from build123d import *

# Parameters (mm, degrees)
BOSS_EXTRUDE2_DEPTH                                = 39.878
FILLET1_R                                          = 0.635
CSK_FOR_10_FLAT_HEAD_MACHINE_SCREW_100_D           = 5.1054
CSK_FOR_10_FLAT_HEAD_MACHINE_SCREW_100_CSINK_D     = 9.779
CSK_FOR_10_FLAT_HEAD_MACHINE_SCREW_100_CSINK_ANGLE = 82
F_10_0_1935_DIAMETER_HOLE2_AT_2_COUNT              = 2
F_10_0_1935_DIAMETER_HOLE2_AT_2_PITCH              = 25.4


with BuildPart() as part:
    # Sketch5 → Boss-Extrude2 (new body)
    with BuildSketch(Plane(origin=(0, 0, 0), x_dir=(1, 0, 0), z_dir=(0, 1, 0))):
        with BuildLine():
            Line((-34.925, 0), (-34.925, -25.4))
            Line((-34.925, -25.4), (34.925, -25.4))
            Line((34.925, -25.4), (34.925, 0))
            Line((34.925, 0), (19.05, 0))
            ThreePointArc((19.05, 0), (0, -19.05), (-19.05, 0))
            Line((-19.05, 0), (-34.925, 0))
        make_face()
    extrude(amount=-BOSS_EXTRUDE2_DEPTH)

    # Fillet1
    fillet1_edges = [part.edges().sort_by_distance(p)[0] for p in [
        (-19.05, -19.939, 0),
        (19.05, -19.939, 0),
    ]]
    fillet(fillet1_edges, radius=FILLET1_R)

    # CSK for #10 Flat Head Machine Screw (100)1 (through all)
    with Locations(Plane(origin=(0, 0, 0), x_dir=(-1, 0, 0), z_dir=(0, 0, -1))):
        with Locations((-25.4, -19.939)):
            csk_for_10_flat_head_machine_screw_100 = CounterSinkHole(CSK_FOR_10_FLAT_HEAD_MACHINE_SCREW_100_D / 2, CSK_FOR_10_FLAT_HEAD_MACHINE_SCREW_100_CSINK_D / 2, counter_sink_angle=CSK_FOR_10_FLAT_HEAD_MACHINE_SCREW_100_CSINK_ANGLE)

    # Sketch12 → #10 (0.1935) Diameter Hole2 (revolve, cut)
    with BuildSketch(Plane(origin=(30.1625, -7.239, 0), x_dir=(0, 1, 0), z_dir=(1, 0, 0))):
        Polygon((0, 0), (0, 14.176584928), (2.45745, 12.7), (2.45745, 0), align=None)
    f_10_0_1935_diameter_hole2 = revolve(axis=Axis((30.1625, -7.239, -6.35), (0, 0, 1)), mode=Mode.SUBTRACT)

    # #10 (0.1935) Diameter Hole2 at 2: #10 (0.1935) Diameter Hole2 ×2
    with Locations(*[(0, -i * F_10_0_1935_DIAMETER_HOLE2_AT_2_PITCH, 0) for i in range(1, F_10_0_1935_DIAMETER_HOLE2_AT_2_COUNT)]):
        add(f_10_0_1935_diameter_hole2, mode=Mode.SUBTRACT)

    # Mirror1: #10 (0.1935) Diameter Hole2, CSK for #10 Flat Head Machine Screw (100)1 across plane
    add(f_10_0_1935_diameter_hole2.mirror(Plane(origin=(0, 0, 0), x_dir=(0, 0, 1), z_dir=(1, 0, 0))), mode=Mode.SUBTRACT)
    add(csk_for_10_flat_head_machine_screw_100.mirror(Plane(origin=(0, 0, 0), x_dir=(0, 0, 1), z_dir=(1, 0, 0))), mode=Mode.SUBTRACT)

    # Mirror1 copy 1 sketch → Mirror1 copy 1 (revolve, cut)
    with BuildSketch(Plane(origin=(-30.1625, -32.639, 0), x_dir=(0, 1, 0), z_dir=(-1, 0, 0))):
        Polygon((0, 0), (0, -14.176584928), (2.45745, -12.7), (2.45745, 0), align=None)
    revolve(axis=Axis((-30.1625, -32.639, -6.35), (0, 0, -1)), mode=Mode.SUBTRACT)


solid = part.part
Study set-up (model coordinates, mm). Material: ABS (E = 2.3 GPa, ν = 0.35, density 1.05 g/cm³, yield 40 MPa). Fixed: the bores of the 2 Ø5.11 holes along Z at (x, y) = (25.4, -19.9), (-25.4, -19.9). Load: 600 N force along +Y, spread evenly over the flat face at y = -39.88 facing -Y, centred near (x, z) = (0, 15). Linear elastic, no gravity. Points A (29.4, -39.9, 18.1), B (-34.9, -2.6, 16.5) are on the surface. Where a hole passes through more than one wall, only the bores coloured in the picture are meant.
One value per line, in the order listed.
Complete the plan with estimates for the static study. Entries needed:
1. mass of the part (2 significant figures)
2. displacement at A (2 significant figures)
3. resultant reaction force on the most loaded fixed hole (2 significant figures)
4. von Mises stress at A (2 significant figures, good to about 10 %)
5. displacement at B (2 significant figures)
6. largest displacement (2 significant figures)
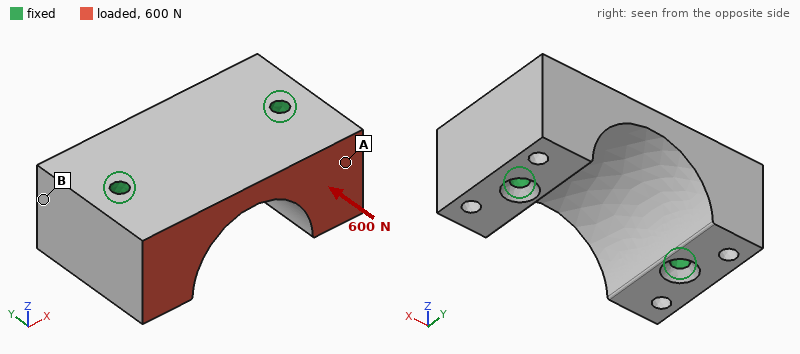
48 g
5.1 µm
300 N
0.56 MPa
2.1 µm
12 µm
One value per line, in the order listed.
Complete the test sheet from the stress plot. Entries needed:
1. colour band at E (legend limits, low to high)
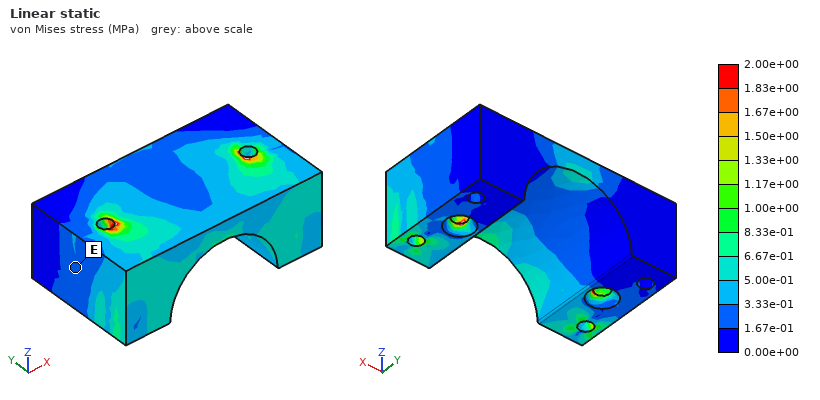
1.67e-01 to 3.33e-01 MPa
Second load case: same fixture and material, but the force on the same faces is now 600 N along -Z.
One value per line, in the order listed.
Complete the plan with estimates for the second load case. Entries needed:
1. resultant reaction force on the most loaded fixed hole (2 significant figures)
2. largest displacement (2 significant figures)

300 N
62 µm
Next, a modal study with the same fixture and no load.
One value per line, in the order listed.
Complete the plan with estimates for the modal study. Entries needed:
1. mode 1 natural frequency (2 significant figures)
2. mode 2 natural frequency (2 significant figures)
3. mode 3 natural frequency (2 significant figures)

5000 Hz
6200 Hz
6300 Hz
